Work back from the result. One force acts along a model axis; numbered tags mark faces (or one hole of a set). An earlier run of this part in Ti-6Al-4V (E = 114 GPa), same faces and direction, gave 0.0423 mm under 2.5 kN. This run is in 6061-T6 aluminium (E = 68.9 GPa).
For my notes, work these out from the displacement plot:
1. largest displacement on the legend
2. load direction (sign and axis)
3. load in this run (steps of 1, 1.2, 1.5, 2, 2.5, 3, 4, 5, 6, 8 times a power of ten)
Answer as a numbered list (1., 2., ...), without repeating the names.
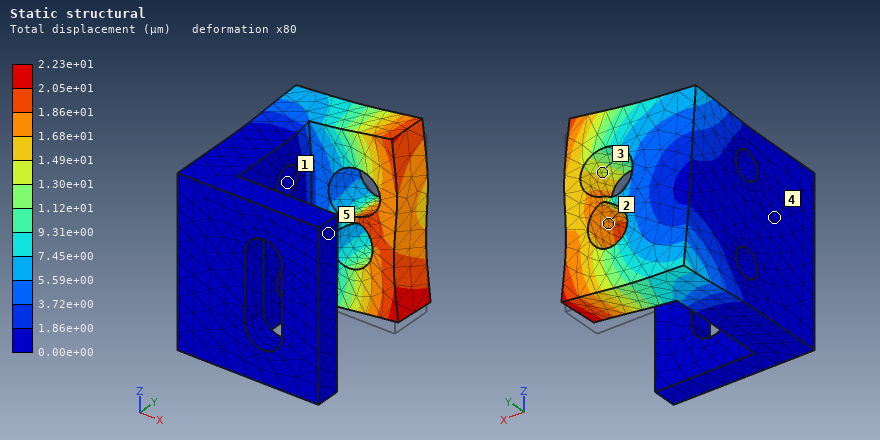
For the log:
1. 2.23e+01 µm
2. +Z
3. 800 N
